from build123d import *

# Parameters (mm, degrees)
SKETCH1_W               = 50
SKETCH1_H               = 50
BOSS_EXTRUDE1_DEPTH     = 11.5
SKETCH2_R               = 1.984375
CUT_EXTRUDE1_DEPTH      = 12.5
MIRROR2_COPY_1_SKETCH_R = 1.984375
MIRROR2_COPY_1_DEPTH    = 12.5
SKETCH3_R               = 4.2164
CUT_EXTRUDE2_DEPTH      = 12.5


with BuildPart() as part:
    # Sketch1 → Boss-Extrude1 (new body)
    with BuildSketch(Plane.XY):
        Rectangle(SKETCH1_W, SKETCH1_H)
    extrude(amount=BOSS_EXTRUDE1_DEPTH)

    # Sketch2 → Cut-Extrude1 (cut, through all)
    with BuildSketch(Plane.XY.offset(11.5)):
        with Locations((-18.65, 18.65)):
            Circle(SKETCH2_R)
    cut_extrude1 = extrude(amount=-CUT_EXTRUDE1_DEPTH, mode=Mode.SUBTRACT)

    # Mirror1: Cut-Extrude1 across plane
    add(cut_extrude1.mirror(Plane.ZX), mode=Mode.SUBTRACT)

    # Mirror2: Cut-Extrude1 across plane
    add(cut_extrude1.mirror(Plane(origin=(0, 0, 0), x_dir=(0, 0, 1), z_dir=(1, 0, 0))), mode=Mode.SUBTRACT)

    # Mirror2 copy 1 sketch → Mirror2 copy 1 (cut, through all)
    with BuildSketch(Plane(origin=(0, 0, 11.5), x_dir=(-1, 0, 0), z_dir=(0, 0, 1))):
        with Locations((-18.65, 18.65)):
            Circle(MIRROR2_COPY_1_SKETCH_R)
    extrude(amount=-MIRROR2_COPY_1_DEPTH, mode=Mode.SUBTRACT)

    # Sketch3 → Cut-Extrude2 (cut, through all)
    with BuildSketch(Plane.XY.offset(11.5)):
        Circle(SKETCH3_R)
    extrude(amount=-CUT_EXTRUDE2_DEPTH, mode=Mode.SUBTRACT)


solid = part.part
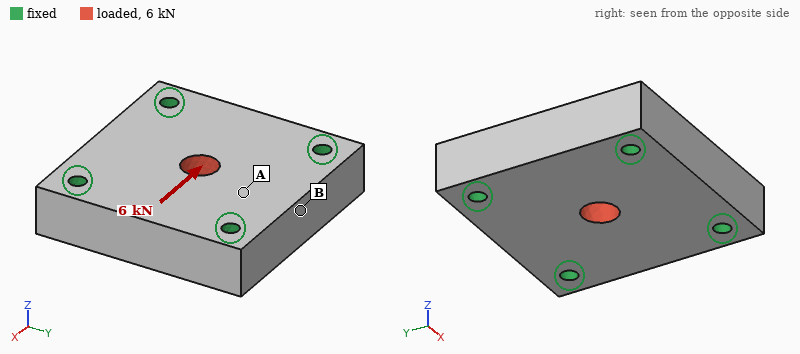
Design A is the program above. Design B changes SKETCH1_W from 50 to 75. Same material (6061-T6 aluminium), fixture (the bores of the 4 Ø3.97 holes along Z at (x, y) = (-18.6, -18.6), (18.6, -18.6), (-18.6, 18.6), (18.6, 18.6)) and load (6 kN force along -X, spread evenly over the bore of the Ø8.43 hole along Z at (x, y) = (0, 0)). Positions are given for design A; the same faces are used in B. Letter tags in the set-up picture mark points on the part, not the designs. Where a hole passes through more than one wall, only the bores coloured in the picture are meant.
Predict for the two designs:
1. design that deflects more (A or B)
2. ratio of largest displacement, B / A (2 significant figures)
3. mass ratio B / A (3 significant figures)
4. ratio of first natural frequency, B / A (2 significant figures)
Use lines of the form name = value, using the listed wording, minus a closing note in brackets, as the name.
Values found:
design that deflects more = A
ratio of largest displacement, B / A = 0.86
mass ratio B / A = 1.52
ratio of first natural frequency, B / A = 0.77
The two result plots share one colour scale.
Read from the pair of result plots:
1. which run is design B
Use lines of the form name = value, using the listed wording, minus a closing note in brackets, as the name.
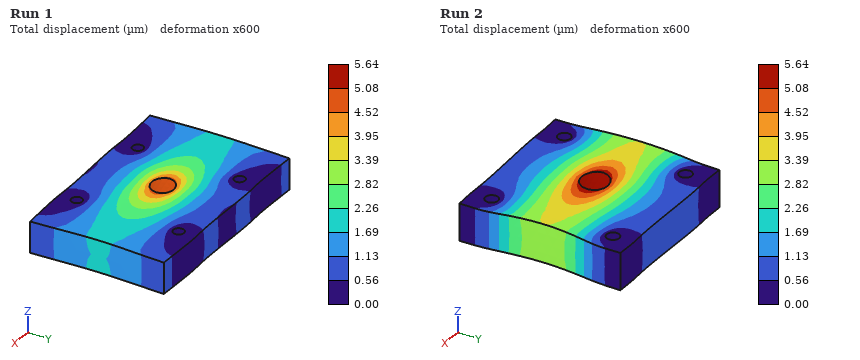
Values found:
which run is design B = Run 1
